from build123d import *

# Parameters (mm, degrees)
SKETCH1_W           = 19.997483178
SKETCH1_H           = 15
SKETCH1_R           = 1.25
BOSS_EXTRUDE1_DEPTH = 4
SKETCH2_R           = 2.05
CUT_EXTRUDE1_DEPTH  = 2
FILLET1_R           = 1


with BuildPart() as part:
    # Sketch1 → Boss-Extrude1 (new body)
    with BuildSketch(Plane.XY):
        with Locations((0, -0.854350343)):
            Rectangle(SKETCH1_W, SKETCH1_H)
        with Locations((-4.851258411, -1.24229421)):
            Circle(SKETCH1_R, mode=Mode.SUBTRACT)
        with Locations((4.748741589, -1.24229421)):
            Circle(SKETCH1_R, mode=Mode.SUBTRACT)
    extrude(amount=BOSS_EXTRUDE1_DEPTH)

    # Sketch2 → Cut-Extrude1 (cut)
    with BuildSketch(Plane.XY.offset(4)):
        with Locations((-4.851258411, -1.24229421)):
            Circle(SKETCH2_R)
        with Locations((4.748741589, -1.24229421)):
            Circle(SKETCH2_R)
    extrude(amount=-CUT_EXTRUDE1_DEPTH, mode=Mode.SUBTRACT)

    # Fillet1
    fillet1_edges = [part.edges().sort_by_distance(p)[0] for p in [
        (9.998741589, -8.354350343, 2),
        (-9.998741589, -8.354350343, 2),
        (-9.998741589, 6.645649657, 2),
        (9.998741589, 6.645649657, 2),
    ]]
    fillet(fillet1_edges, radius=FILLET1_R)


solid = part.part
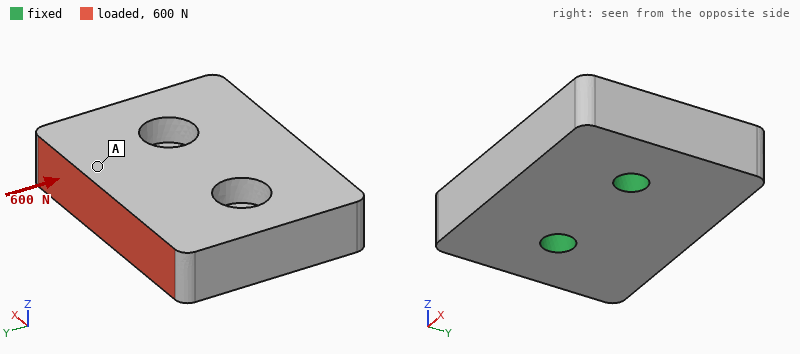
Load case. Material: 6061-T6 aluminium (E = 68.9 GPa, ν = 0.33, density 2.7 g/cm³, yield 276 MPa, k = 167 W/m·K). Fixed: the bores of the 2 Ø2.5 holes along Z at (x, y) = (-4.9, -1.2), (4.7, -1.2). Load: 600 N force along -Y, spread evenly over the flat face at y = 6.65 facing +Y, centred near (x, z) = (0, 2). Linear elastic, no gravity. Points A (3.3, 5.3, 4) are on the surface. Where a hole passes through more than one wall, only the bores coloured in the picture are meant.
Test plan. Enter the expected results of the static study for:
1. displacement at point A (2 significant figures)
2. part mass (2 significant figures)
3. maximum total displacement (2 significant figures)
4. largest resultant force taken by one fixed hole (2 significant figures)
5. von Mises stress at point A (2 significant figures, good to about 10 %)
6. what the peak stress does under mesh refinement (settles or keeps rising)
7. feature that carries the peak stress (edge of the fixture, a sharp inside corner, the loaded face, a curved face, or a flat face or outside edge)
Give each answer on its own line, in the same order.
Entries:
4.6 µm
3.0 g
5.3 µm
300 N
8.2 MPa
keeps rising
edge of the fixture
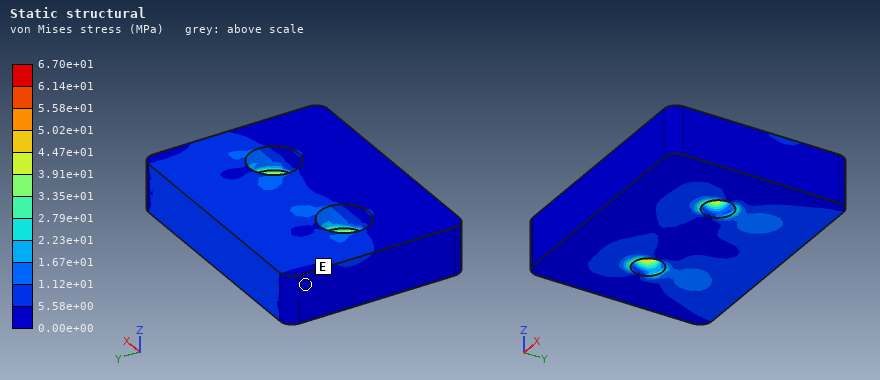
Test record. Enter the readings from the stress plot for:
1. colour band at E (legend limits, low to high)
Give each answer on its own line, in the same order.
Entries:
0.00e+00 to 5.58e+00 MPa
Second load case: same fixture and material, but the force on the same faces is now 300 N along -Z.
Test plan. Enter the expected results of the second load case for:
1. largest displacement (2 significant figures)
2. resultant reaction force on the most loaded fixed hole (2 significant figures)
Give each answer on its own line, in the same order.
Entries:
22 µm
150 N
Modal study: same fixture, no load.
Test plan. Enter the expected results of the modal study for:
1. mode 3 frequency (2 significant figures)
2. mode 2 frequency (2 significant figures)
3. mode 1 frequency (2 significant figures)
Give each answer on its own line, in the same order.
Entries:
44 kHz
38 kHz
22 kHz
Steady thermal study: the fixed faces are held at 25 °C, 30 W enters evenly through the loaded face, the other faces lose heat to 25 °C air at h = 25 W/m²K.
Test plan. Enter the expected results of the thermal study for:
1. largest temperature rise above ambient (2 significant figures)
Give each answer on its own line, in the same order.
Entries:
23 K
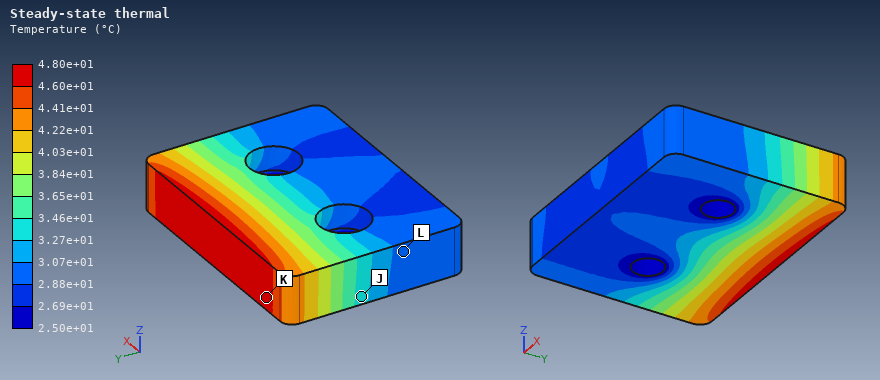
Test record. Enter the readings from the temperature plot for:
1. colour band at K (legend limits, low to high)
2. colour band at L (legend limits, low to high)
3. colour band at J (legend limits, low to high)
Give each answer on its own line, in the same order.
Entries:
4.60e+01 to 4.80e+01 °C
2.88e+01 to 3.07e+01 °C
3.27e+01 to 3.46e+01 °C
